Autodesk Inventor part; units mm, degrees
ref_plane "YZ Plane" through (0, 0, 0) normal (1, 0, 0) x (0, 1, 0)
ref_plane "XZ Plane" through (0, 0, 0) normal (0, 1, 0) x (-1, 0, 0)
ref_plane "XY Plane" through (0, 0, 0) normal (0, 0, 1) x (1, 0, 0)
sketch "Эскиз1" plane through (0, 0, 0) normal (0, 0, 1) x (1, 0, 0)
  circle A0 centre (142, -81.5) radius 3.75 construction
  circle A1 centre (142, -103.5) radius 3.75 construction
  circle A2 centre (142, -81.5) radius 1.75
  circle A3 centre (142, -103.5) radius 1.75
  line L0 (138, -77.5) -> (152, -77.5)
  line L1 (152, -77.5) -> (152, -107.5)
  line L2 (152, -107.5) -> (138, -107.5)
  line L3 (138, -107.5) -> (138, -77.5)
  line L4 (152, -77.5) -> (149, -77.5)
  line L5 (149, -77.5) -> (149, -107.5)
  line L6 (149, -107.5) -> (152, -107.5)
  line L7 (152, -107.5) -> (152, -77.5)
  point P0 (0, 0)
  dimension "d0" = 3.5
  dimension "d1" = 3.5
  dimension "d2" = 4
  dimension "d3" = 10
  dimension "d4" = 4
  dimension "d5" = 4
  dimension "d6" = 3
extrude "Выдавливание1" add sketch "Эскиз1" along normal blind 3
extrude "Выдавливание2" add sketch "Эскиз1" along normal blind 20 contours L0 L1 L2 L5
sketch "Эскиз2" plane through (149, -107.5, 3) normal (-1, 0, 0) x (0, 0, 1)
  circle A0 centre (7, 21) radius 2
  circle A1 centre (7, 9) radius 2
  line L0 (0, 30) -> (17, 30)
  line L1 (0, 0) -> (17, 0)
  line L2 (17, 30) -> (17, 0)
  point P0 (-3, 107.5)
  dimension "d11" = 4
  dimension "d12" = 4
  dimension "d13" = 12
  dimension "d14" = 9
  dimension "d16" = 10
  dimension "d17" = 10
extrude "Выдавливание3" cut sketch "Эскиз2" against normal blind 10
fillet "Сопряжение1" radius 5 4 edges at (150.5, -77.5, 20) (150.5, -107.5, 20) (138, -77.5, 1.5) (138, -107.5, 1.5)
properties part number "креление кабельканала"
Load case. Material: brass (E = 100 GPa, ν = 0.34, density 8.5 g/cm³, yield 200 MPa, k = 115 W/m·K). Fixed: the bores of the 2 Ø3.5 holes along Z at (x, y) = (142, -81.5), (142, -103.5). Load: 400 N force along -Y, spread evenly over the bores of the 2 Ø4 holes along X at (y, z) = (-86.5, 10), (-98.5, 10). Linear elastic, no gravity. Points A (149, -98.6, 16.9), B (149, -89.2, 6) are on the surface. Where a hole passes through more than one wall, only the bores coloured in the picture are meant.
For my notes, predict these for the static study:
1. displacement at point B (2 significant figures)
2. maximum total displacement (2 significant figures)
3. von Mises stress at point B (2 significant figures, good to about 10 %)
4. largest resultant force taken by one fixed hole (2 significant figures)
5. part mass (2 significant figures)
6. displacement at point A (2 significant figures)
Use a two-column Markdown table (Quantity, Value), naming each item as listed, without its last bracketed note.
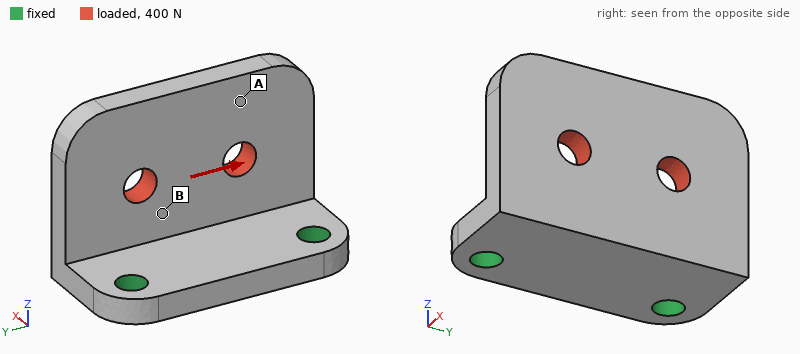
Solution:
| Quantity | Value |
|---|---|
| displacement at point B | 4.6 µm |
| maximum total displacement | 16 µm |
| von Mises stress at point B | 19 MPa |
| largest resultant force taken by one fixed hole | 280 N |
| part mass | 22 g |
| displacement at point A | 12 µm |
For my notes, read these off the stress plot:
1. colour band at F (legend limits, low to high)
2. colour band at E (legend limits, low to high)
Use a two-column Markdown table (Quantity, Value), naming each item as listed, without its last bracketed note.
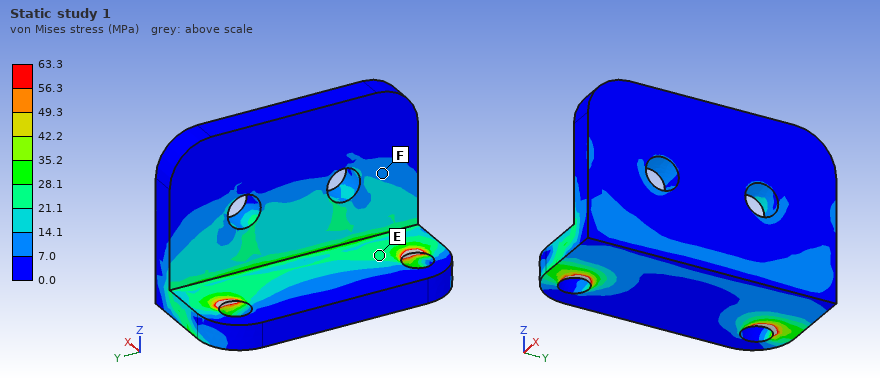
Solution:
| Quantity | Value |
|---|---|
| colour band at F | 7.0 to 14.1 MPa |
| colour band at E | 21.1 to 28.1 MPa |
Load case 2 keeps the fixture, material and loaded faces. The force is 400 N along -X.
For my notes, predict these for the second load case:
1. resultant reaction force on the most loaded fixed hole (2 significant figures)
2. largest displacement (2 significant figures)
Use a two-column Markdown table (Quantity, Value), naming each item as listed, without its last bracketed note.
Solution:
| Quantity | Value |
|---|---|
| resultant reaction force on the most loaded fixed hole | 220 N |
| largest displacement | 0.11 mm |
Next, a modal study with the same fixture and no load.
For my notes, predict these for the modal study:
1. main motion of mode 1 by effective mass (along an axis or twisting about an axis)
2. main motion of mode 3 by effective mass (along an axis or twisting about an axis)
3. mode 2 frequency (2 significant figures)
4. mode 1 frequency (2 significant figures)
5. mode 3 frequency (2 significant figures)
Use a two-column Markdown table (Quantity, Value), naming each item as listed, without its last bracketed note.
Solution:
| Quantity | Value |
|---|---|
| main motion of mode 1 by effective mass | along X |
| main motion of mode 3 by effective mass | along Y |
| mode 2 frequency | 6200 Hz |
| mode 1 frequency | 3000 Hz |
| mode 3 frequency | 9400 Hz |
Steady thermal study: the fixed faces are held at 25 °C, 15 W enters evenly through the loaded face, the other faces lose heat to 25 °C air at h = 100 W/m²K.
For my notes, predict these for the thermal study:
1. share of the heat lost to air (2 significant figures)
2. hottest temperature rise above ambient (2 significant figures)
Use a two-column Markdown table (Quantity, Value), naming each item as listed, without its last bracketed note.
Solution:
| Quantity | Value |
|---|---|
| share of the heat lost to air | 18 % |
| hottest temperature rise above ambient | 25 K |
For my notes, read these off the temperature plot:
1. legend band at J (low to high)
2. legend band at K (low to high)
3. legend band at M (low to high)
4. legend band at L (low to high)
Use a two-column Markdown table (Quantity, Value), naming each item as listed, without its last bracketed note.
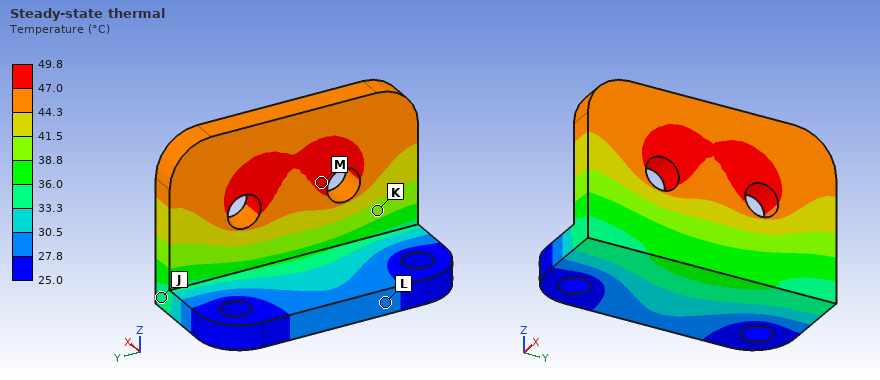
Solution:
| Quantity | Value |
|---|---|
| legend band at J | 33.3 to 36.0 °C |
| legend band at K | 38.8 to 41.5 °C |
| legend band at M | 47.0 to 49.8 °C |
| legend band at L | 27.8 to 30.5 °C |
